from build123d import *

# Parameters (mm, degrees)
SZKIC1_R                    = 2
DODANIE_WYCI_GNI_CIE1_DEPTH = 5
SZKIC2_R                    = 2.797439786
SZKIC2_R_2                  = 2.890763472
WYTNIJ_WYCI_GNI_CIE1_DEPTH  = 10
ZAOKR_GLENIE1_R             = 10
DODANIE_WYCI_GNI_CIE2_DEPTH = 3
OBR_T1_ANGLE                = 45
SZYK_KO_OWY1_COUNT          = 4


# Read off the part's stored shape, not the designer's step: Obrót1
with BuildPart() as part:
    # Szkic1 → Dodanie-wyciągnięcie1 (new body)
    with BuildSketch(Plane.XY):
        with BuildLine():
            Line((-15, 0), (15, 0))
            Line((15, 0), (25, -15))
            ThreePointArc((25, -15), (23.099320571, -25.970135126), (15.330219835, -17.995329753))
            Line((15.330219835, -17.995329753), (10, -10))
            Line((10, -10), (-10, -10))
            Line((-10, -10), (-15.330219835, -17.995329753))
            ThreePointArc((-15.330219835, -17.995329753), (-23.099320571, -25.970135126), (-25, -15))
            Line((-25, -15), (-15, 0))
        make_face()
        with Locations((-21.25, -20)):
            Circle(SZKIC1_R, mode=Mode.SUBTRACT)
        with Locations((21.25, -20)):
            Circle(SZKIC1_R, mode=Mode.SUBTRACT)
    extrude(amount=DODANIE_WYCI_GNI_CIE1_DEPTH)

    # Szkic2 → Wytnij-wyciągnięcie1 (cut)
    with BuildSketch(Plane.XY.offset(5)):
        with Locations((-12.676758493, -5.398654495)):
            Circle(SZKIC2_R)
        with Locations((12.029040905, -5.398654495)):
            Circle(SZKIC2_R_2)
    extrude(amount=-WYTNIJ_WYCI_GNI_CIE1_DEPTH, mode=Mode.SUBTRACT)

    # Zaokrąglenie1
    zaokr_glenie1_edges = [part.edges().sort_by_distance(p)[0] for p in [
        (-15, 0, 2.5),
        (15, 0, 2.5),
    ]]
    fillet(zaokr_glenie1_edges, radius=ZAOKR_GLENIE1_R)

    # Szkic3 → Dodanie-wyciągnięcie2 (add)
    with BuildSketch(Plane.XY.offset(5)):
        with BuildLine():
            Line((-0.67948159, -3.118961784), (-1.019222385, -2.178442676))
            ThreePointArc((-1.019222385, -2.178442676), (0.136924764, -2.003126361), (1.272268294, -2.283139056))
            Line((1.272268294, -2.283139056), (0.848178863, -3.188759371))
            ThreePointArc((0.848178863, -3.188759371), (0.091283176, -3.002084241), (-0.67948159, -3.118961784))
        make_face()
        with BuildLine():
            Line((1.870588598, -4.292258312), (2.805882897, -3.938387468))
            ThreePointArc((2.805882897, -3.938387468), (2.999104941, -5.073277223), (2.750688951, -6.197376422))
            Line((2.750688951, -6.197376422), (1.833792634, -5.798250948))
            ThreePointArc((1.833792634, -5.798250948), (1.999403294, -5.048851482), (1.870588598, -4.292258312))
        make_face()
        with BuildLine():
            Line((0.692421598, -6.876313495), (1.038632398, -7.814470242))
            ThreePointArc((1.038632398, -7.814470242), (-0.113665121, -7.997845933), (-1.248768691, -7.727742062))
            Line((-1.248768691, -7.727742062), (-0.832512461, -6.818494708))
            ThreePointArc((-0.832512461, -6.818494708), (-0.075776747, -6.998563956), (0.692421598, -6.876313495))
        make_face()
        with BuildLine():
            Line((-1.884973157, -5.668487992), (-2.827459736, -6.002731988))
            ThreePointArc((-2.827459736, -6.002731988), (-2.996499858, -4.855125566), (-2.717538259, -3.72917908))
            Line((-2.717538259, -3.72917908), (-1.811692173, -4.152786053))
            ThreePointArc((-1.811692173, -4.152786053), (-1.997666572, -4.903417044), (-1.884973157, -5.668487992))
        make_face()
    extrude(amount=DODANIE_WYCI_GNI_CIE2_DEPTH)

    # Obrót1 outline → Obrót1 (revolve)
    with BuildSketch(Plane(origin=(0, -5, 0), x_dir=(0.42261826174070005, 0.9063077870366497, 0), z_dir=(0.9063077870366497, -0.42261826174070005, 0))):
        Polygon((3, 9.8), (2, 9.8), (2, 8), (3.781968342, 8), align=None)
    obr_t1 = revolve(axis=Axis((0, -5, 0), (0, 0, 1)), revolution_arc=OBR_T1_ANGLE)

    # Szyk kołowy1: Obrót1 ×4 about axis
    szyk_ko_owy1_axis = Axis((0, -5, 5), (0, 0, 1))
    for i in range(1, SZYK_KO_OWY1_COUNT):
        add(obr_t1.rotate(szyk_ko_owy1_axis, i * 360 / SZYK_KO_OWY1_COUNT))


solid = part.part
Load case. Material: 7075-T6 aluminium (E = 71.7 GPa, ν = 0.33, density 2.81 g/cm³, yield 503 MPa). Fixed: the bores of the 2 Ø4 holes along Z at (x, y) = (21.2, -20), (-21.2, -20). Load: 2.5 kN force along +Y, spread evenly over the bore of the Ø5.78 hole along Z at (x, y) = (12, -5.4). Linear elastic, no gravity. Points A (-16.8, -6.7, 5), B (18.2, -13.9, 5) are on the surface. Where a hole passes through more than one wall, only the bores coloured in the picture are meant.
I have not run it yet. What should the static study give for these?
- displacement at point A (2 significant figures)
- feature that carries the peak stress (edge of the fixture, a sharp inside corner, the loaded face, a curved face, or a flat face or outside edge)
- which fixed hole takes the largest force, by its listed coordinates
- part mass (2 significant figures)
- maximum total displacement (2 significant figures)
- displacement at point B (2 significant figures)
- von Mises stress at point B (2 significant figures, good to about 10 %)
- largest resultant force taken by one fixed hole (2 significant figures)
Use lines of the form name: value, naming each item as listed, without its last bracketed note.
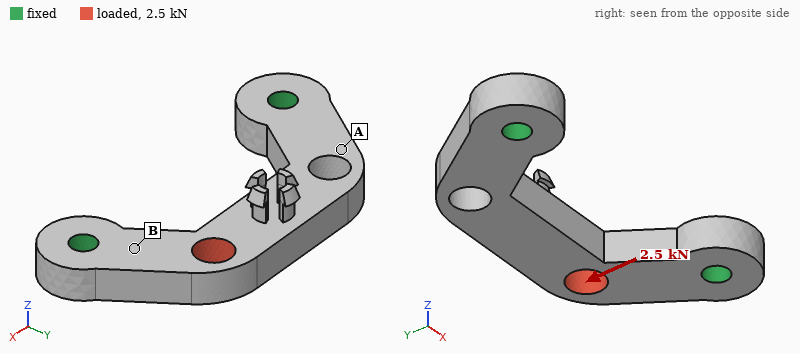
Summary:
displacement at point A: 7.5 µm
feature that carries the peak stress: the loaded face
which fixed hole takes the largest force, by its listed coordinates: (21.2, -20)
part mass: 9.2 g
maximum total displacement: 31 µm
displacement at point B: 7.3 µm
von Mises stress at point B: 52 MPa
largest resultant force taken by one fixed hole: 2.2 kN
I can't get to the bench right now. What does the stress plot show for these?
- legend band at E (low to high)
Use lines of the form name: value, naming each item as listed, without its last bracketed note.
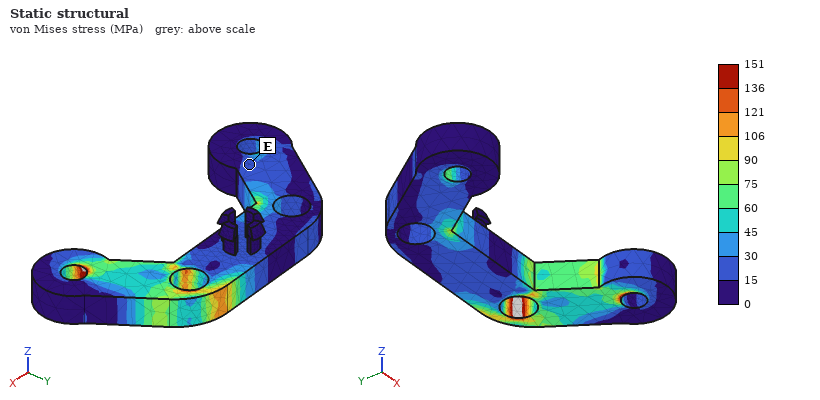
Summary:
legend band at E: 15 to 30 MPa
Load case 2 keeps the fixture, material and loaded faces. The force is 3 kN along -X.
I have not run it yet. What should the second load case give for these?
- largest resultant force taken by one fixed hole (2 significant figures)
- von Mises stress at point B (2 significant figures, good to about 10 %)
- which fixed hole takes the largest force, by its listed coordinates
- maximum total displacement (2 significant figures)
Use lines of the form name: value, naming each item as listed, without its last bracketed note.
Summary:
largest resultant force taken by one fixed hole: 1.8 kN
von Mises stress at point B: 67 MPa
which fixed hole takes the largest force, by its listed coordinates: (21.2, -20)
maximum total displacement: 44 µm
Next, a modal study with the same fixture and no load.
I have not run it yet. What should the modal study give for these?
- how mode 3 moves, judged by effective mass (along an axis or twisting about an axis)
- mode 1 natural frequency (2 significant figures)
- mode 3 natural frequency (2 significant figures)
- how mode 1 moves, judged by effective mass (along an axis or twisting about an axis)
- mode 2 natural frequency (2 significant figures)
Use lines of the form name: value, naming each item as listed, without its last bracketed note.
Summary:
how mode 3 moves, judged by effective mass: along X
mode 1 natural frequency: 6800 Hz
mode 3 natural frequency: 21 kHz
how mode 1 moves, judged by effective mass: along Z
mode 2 natural frequency: 16 kHz
